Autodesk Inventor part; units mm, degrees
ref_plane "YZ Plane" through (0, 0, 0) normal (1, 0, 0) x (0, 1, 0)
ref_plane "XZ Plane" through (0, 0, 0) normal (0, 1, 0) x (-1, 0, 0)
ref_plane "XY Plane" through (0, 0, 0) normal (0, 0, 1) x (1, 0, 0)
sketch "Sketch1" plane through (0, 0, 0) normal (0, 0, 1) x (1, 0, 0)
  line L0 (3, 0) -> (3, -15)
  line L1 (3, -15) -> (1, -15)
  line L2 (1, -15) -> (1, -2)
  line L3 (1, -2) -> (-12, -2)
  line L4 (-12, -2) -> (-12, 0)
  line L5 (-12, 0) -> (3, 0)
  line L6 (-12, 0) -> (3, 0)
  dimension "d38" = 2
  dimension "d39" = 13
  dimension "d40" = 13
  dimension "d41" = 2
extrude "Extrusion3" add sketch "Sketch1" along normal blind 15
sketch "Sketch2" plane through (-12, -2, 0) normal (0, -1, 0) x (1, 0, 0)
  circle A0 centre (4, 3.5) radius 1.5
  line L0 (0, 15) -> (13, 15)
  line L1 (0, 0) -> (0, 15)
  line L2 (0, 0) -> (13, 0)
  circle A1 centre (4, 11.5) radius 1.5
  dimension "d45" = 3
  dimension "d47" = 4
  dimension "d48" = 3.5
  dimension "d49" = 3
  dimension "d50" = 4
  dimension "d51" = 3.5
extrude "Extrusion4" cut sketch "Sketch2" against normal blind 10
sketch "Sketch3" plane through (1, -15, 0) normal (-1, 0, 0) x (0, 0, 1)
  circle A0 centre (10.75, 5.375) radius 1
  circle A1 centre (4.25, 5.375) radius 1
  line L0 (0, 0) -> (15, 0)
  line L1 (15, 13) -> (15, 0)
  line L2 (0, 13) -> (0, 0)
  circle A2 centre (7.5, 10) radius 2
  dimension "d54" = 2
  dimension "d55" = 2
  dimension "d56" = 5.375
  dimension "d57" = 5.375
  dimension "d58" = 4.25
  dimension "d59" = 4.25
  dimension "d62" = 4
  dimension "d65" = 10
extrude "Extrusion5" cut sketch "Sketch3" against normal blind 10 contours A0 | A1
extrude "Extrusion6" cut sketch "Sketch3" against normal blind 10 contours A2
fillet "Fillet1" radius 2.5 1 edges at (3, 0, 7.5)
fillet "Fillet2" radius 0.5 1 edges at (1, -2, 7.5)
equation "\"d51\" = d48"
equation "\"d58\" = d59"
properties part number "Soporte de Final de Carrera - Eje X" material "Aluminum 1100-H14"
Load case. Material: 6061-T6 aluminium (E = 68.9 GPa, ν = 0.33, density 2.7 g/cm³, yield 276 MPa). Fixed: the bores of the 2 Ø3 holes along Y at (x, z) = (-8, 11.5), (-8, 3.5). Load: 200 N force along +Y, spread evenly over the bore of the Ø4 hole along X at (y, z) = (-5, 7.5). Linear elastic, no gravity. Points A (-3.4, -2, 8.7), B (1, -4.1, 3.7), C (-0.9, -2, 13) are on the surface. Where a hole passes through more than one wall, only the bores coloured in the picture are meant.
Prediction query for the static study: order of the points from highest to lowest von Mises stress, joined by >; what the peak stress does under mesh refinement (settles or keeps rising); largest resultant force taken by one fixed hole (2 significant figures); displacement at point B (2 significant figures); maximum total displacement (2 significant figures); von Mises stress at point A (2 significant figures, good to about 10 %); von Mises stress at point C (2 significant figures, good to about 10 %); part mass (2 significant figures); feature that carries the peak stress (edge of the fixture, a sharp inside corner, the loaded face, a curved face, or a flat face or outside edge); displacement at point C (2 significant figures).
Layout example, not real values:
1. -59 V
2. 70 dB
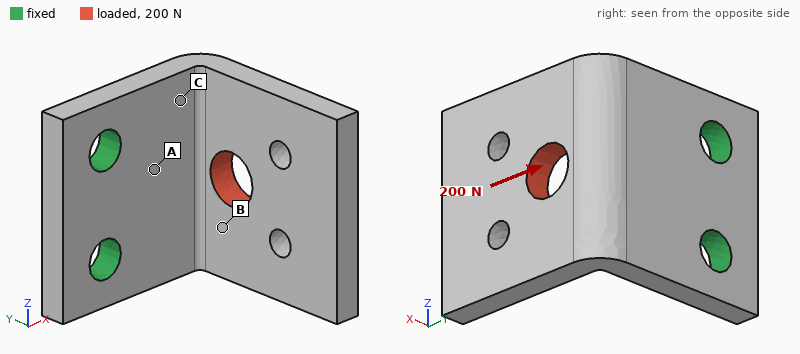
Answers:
1. A > C > B
2. keeps rising
3. 100 N
4. 0.070 mm
5. 0.18 mm
6. 94 MPa
7. 54 MPa
8. 2.0 g
9. edge of the fixture
10. 0.041 mm
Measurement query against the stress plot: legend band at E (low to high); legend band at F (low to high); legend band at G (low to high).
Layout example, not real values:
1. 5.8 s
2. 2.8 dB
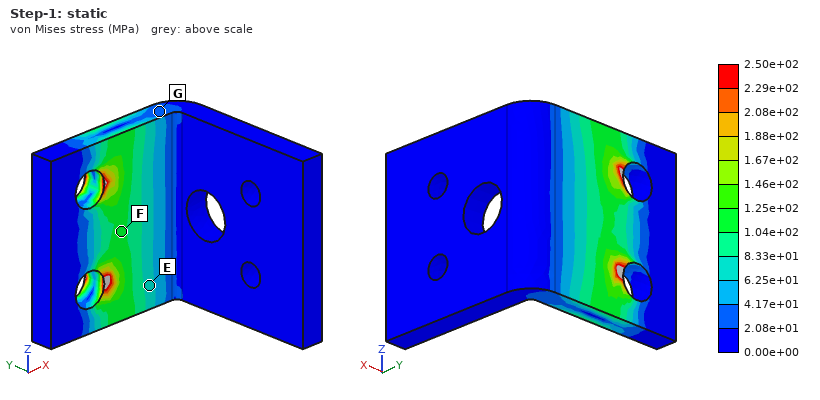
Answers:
1. 6.25e+01 to 8.33e+01 MPa
2. 1.04e+02 to 1.25e+02 MPa
3. 2.08e+01 to 4.17e+01 MPa
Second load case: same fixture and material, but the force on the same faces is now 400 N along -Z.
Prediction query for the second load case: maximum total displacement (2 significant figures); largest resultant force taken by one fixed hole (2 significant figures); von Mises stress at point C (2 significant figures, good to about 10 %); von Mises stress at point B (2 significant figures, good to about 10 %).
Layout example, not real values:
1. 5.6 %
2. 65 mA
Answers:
1. 0.13 mm
2. 450 N
3. 110 MPa
4. 63 MPa
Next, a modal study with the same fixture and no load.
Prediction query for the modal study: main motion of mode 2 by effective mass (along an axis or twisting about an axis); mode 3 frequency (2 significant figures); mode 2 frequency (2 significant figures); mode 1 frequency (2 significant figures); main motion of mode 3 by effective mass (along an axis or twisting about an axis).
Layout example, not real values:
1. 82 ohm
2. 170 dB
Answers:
1. along Z
2. 12 kHz
3. 7200 Hz
4. 4100 Hz
5. along Y
